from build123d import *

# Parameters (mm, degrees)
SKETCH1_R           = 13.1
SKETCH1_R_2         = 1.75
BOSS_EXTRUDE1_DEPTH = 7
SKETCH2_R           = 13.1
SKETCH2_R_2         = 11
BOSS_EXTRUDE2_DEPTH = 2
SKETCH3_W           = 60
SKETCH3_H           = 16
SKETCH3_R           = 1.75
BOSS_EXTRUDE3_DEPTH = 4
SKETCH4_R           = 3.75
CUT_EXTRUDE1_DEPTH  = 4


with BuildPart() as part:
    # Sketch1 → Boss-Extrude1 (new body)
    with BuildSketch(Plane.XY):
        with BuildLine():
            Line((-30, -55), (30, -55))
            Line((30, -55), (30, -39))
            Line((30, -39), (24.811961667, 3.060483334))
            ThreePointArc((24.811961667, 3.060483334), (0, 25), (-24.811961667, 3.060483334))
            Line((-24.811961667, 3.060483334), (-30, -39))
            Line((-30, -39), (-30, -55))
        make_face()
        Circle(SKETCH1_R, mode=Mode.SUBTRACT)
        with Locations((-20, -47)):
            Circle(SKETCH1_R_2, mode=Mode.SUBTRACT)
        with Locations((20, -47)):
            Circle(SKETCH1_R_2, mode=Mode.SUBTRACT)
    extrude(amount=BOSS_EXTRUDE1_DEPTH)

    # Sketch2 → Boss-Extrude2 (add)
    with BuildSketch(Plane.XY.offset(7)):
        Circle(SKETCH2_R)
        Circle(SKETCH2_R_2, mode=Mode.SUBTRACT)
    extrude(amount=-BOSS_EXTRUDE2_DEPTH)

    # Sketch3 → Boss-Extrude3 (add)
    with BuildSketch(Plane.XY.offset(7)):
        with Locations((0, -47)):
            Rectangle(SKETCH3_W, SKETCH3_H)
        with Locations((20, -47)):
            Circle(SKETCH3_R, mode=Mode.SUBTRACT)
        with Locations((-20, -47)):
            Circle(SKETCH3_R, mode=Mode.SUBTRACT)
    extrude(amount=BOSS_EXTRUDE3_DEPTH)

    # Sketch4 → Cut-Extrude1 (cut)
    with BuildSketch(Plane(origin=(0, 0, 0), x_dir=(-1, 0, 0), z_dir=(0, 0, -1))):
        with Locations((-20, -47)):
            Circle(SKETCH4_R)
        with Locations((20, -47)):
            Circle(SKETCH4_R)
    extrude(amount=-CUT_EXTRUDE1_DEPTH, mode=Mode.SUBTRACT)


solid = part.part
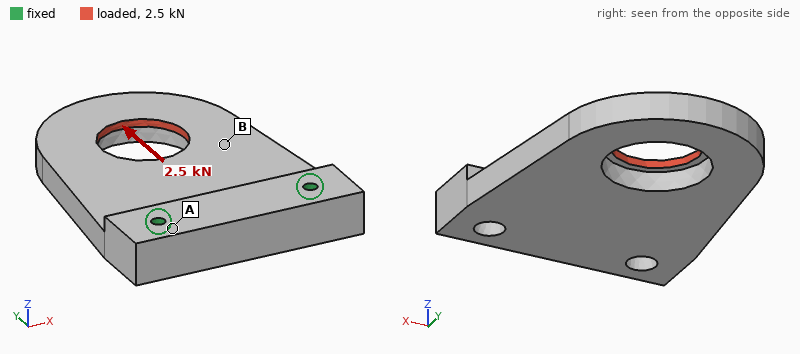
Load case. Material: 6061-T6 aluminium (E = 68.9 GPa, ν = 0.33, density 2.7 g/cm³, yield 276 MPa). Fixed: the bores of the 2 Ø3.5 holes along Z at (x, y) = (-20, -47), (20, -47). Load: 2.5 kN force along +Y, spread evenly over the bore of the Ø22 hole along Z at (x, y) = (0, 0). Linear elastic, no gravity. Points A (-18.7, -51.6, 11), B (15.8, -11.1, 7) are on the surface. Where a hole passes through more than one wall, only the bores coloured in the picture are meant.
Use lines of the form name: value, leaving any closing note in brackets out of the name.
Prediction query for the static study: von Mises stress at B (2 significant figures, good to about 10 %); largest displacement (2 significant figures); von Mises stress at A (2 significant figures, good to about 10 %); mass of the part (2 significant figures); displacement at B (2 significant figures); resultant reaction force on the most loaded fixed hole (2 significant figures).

von Mises stress at B: 23 MPa
largest displacement: 0.11 mm
von Mises stress at A: 5.2 MPa
mass of the part: 77 g
displacement at B: 0.021 mm
resultant reaction force on the most loaded fixed hole: 1.3 kN
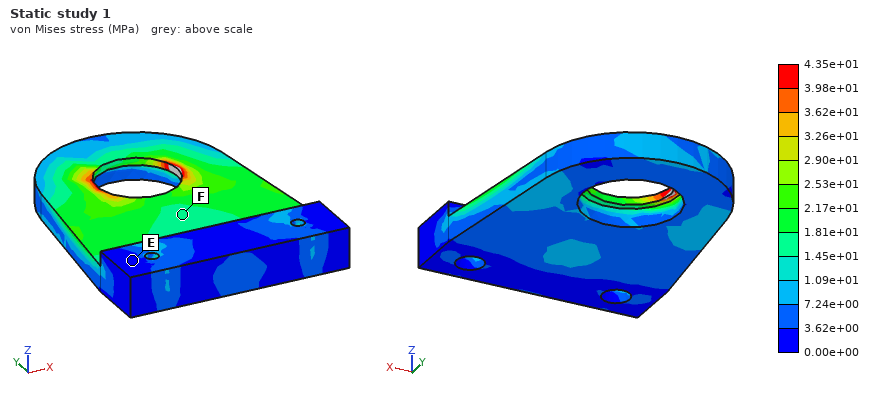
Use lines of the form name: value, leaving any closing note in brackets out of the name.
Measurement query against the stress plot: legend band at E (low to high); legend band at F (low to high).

legend band at E: 0.00e+00 to 3.62e+00 MPa
legend band at F: 1.45e+01 to 1.81e+01 MPa
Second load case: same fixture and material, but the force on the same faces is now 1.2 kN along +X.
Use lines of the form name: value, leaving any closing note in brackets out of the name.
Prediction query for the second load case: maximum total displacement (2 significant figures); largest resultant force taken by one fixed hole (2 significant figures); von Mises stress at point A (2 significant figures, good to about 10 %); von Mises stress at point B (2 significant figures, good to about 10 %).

maximum total displacement: 38 µm
largest resultant force taken by one fixed hole: 1.5 kN
von Mises stress at point A: 8.9 MPa
von Mises stress at point B: 11 MPa
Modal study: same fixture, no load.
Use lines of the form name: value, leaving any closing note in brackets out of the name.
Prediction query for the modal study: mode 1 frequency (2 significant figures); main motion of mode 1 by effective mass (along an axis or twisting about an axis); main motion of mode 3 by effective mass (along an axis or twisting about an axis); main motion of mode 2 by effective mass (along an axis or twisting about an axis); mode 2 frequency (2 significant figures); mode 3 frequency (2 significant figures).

mode 1 frequency: 1400 Hz
main motion of mode 1 by effective mass: along Z
main motion of mode 3 by effective mass: along Z
main motion of mode 2 by effective mass: twisting about Y
mode 2 frequency: 4100 Hz
mode 3 frequency: 6100 Hz
